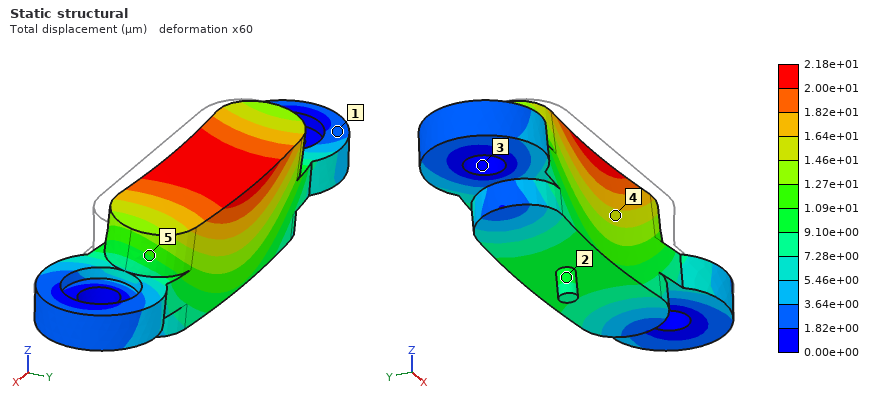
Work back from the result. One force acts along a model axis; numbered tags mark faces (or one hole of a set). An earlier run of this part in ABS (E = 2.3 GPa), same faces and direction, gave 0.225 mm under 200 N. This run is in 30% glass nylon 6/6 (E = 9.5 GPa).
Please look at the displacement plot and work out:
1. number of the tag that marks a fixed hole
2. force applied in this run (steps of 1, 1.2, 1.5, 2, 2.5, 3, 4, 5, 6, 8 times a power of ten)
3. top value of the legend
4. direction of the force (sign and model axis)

3
80 N
2.18e+01 µm
+Y
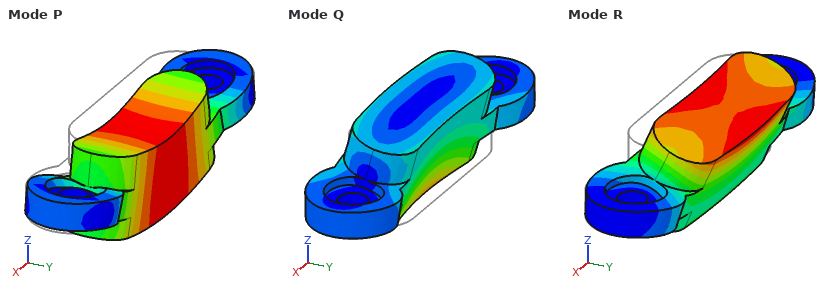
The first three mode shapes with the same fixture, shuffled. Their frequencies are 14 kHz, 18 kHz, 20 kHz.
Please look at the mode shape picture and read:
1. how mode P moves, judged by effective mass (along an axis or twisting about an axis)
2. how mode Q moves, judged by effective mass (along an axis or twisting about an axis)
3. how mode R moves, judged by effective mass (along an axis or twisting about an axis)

along Z
along Y
along Y
